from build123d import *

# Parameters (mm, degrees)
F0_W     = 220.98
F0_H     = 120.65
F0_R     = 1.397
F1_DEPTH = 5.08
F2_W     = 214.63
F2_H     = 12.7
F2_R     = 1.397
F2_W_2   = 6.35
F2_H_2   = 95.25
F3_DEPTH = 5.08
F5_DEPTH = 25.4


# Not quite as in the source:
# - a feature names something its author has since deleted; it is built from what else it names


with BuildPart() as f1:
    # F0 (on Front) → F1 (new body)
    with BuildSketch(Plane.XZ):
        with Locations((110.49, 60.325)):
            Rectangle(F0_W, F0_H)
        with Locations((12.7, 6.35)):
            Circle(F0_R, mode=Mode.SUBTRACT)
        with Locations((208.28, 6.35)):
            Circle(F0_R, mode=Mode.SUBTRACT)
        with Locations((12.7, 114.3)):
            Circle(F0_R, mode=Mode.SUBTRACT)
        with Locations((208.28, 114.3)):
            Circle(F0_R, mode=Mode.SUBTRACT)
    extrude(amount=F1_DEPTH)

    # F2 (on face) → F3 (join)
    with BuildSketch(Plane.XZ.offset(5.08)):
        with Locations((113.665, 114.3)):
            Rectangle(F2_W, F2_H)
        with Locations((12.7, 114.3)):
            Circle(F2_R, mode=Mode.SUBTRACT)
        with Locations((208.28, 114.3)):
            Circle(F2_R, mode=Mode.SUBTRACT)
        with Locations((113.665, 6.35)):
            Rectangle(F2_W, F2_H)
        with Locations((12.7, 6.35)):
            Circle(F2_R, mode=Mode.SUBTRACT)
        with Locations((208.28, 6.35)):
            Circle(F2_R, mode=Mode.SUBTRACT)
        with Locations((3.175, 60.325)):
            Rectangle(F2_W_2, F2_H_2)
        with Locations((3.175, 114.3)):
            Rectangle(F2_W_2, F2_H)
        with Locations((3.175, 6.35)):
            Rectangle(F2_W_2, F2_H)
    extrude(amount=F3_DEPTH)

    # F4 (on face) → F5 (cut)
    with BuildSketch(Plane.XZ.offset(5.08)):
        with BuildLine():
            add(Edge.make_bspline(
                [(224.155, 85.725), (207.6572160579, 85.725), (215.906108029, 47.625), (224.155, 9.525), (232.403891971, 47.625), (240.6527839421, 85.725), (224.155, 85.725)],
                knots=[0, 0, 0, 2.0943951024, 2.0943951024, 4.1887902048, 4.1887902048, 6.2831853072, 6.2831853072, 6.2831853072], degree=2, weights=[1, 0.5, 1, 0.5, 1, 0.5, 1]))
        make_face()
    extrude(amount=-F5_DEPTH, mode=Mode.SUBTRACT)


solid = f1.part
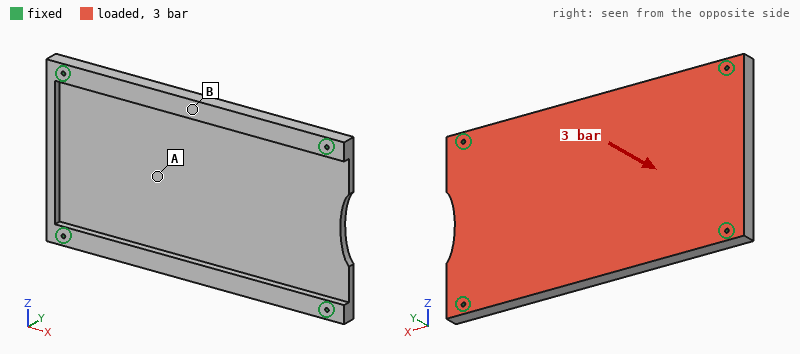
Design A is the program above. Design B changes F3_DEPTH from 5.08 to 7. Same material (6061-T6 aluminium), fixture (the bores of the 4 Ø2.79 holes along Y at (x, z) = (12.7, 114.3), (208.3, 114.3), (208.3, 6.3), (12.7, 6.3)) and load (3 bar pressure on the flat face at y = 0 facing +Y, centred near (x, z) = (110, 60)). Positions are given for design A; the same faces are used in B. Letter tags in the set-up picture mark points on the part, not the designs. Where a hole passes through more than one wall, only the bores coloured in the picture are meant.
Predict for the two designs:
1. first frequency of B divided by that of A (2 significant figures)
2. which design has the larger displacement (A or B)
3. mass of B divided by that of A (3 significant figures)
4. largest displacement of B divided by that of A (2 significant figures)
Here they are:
1.2
A
1.07
0.74
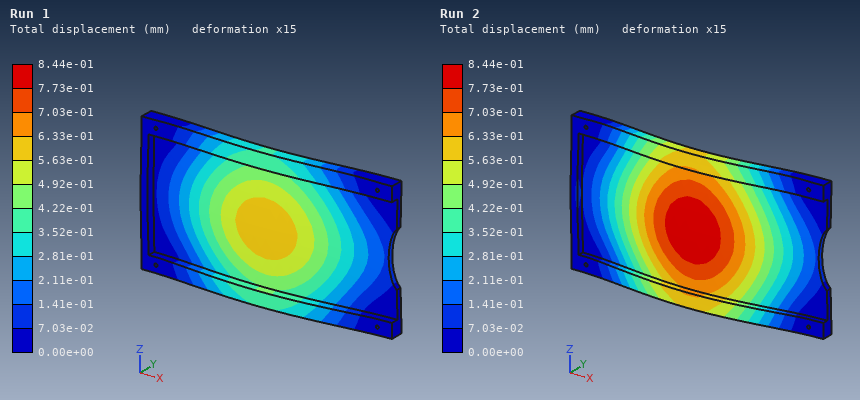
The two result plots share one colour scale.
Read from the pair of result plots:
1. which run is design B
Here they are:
Run 1
